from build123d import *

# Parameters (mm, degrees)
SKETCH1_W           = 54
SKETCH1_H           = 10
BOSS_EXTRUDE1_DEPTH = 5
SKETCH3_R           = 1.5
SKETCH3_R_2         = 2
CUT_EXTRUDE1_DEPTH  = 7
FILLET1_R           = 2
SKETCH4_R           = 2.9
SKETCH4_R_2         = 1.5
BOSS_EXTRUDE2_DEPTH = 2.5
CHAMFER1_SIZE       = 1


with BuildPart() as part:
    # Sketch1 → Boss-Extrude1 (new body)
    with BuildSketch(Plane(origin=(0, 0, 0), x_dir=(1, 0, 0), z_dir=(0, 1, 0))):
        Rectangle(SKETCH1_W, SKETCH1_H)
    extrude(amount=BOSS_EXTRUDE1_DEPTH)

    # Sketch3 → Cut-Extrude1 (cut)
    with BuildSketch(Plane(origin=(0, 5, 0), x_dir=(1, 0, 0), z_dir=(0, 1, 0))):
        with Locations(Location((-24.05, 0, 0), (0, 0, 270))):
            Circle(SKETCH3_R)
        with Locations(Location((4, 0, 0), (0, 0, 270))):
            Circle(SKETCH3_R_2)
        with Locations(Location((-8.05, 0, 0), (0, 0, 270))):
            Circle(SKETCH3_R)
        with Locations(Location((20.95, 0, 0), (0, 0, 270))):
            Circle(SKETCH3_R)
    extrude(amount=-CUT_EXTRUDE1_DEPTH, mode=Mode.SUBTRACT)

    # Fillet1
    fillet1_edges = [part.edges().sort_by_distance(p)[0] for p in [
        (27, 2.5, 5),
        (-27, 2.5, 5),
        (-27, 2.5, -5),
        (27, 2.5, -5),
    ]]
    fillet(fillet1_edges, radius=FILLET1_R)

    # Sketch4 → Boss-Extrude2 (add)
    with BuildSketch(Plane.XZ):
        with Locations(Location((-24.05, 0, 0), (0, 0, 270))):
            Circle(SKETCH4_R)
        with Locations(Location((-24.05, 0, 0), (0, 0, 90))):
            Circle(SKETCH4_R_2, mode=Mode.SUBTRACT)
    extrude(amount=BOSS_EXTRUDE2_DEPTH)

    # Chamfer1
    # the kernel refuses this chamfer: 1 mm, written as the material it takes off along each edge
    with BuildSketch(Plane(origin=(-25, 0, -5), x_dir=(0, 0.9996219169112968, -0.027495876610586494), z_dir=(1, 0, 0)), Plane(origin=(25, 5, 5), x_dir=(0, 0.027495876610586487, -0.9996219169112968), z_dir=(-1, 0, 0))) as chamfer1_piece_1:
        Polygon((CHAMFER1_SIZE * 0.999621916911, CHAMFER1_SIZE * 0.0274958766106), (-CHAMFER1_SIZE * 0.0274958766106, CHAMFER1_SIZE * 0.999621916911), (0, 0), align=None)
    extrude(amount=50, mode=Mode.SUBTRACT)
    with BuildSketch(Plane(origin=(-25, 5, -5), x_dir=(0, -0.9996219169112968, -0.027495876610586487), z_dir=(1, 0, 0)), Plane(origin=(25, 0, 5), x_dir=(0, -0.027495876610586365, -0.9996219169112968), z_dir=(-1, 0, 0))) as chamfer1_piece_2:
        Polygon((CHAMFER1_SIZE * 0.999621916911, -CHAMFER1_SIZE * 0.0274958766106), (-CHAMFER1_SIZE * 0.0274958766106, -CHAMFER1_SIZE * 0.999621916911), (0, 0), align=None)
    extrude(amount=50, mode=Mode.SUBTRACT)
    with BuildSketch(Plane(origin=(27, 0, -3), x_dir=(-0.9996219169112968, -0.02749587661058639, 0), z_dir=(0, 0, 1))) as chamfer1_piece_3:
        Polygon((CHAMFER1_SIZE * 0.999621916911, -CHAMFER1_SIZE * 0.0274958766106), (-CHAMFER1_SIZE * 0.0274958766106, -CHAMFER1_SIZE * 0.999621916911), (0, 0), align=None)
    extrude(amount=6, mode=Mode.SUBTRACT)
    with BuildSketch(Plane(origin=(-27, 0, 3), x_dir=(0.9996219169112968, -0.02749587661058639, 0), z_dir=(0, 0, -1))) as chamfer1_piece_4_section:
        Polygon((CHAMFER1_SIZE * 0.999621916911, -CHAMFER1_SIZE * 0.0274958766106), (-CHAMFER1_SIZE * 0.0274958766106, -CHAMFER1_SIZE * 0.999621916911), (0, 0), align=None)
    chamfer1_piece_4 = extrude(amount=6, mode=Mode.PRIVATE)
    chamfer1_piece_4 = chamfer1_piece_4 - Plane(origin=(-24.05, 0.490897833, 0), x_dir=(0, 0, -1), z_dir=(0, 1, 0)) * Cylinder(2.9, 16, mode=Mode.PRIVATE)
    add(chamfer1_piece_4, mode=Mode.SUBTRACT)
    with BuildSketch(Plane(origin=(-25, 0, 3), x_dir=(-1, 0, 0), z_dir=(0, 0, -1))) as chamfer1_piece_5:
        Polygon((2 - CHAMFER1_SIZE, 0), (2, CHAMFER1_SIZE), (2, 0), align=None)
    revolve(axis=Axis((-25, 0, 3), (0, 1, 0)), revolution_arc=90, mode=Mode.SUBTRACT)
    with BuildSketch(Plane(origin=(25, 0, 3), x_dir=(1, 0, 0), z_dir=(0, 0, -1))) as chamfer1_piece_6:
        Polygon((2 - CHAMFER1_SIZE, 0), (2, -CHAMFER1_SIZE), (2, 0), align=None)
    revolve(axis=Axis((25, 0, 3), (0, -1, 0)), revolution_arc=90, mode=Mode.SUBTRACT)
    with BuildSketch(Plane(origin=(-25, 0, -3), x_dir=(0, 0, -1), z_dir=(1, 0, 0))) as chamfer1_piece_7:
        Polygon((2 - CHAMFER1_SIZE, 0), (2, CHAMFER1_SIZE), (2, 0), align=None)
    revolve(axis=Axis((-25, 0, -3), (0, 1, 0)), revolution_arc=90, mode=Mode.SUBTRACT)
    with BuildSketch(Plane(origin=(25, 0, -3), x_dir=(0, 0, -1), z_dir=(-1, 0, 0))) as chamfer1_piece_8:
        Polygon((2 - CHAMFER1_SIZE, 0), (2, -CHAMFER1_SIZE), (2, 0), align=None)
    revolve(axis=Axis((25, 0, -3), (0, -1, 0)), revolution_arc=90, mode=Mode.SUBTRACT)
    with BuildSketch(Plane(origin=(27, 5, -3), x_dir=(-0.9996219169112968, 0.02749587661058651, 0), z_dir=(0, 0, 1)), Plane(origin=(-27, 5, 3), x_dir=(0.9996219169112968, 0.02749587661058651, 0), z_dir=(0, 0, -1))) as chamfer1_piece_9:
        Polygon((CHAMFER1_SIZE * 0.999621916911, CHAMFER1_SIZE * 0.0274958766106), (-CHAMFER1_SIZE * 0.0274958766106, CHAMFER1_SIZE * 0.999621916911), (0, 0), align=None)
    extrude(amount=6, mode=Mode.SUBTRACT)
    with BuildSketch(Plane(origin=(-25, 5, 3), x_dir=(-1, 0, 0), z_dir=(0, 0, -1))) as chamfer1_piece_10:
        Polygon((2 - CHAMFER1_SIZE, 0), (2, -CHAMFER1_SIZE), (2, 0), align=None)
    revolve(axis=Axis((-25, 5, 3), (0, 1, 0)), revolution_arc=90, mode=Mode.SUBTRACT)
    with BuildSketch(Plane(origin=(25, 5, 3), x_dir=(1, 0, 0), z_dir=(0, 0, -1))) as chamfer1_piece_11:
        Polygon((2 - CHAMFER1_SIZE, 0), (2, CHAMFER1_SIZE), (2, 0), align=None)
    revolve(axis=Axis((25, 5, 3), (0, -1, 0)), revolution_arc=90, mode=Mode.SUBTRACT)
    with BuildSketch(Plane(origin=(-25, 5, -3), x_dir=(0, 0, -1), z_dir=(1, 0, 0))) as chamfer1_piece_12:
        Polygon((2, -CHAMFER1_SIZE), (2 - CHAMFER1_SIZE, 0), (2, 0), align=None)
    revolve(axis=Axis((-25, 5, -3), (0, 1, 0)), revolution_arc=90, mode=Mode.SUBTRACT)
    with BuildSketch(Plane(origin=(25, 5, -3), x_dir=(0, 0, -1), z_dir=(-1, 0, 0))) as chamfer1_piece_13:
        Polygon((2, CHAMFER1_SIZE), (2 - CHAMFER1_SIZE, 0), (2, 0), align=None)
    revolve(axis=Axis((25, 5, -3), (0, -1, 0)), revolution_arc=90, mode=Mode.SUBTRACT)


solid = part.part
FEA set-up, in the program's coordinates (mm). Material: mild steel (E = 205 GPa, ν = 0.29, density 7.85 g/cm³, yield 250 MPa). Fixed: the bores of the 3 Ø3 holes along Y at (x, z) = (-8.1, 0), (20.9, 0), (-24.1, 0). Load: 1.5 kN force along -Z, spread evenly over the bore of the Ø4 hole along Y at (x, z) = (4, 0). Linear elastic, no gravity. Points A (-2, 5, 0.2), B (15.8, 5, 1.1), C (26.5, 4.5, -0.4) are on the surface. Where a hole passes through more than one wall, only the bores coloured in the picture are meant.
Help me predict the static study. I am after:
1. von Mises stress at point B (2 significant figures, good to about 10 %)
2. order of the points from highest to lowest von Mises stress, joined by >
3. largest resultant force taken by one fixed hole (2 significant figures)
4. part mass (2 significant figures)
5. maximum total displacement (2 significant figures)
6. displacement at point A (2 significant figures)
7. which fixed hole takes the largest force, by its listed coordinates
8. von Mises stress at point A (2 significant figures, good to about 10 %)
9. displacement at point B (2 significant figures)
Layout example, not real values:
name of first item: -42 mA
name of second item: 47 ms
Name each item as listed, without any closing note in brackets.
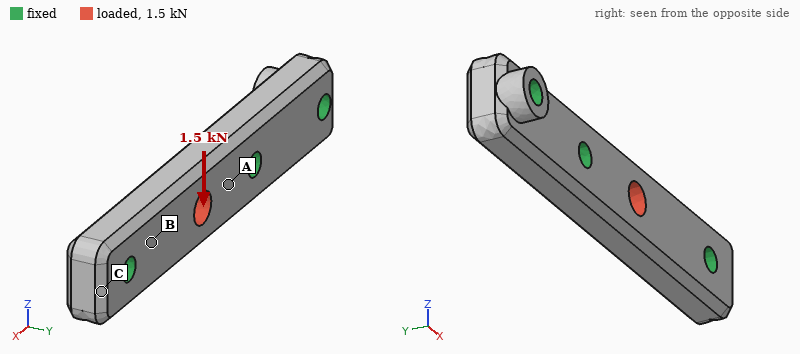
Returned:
von Mises stress at point B: 30 MPa
order of the points from highest to lowest von Mises stress, joined by >: A > B > C
largest resultant force taken by one fixed hole: 1.1 kN
part mass: 19 g
maximum total displacement: 6.8 µm
displacement at point A: 3.1 µm
which fixed hole takes the largest force, by its listed coordinates: (-8.1, 0)
von Mises stress at point A: 51 MPa
displacement at point B: 2.2 µm
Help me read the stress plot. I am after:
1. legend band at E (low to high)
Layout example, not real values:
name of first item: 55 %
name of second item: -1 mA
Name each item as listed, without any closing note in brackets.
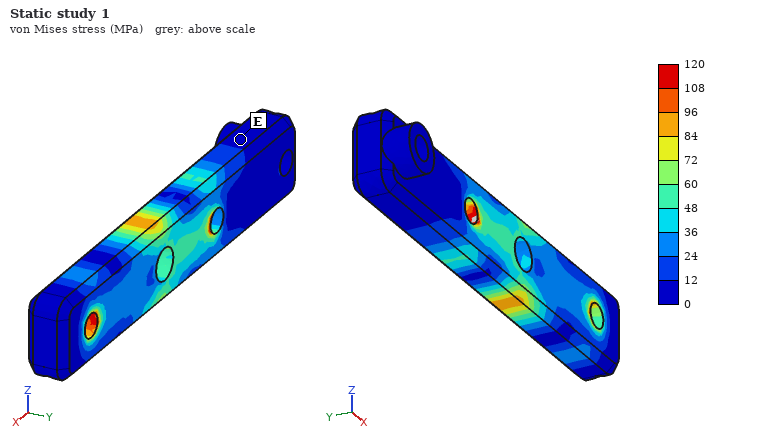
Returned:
legend band at E: 0 to 12 MPa
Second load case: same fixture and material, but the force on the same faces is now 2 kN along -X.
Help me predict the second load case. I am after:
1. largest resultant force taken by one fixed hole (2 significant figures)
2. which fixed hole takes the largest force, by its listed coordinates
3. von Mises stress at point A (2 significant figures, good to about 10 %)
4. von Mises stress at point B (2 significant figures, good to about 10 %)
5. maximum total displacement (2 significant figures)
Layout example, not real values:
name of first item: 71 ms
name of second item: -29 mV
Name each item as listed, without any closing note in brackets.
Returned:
largest resultant force taken by one fixed hole: 1.1 kN
which fixed hole takes the largest force, by its listed coordinates: (-8.1, 0)
von Mises stress at point A: 31 MPa
von Mises stress at point B: 22 MPa
maximum total displacement: 1.6 µm
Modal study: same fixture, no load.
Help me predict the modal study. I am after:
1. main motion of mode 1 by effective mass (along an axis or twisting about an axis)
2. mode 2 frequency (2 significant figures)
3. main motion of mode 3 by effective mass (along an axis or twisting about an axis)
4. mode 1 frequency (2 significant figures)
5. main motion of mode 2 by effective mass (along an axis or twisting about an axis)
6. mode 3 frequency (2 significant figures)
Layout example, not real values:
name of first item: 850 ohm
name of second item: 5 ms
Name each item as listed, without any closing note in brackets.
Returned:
main motion of mode 1 by effective mass: along Y
mode 2 frequency: 35 kHz
main motion of mode 3 by effective mass: twisting about X
mode 1 frequency: 27 kHz
main motion of mode 2 by effective mass: along Z
mode 3 frequency: 44 kHz
